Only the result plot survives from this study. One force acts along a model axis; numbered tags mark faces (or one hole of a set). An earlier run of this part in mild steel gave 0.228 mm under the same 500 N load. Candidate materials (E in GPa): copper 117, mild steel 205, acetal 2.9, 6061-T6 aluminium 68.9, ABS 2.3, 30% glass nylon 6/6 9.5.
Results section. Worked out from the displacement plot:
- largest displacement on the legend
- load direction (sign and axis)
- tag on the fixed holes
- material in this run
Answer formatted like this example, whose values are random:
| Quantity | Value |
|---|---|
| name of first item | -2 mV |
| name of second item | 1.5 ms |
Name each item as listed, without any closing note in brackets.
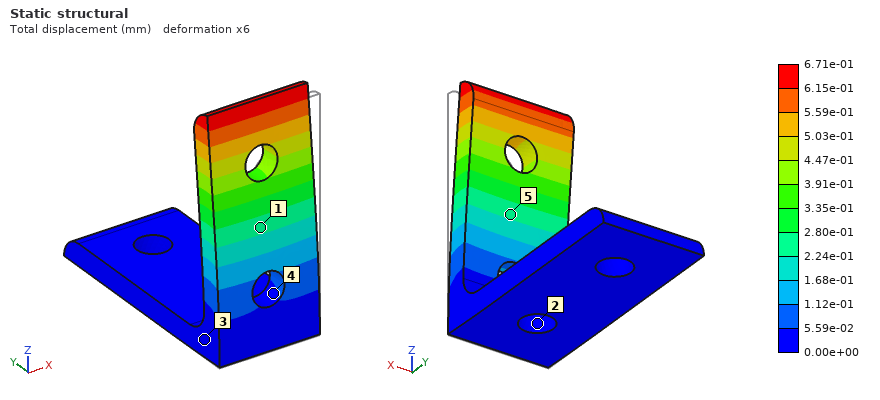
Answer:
| Quantity | Value |
|---|---|
| largest displacement on the legend | 6.71e-01 mm |
| load direction | +Y |
| tag on the fixed holes | 2 |
| material in this run | 6061-T6 aluminium |
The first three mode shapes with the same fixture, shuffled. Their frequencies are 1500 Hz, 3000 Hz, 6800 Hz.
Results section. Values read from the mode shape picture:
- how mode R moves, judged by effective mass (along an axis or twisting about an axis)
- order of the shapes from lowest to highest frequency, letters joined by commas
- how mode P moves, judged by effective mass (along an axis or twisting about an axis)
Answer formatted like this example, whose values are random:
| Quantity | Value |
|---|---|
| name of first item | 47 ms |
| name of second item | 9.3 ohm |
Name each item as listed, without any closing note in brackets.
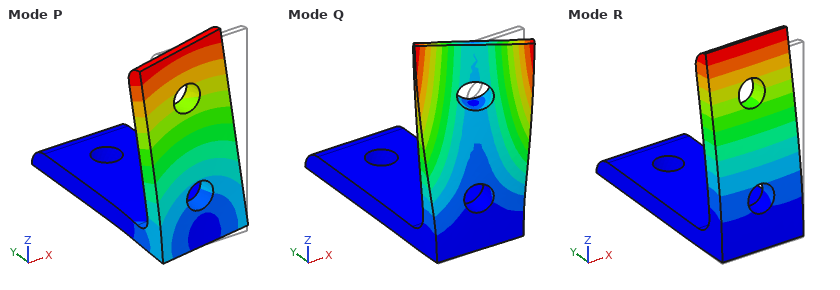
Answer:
| Quantity | Value |
|---|---|
| how mode R moves, judged by effective mass | along Y |
| order of the shapes from lowest to highest frequency, letters joined by commas | R, P, Q |
| how mode P moves, judged by effective mass | along X |
